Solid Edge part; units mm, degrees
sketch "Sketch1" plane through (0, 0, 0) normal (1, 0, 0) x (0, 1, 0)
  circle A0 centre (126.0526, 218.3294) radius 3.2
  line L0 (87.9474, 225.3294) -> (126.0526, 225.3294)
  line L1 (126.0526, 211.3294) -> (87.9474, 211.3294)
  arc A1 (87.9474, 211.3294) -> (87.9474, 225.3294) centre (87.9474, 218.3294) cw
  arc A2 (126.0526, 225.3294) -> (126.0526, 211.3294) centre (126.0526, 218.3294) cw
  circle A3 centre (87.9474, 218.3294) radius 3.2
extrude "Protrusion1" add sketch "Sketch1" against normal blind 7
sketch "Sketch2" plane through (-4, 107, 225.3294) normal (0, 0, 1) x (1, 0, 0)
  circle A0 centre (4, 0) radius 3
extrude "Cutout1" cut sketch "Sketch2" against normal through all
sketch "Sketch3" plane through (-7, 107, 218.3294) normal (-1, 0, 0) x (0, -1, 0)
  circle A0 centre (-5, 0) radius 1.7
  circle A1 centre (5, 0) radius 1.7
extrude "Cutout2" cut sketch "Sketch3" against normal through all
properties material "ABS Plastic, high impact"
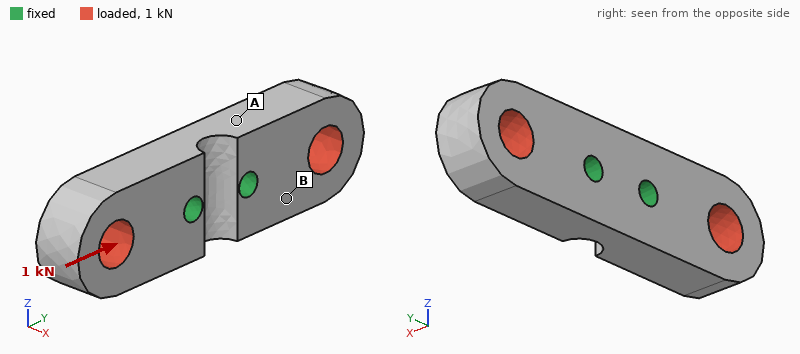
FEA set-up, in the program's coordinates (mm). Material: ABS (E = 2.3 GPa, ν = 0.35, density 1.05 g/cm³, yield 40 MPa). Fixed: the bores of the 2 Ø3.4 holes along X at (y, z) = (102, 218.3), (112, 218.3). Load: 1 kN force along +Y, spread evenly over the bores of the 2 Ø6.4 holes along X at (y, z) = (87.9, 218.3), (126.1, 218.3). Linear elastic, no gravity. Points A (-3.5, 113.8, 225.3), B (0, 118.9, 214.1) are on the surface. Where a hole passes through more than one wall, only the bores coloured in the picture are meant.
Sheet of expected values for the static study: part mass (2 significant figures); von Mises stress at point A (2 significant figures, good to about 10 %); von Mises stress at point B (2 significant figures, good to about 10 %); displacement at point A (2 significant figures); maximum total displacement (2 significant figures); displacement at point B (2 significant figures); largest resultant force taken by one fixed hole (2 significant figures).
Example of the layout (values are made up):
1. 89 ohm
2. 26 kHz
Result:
1. 4.2 g
2. 2.5 MPa
3. 5.5 MPa
4. 18 µm
5. 69 µm
6. 23 µm
7. 500 N
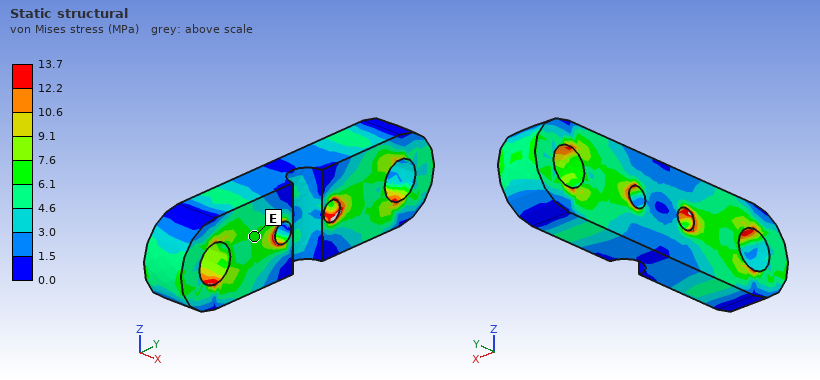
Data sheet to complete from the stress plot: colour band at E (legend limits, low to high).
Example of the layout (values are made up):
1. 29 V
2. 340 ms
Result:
1. 6.1 to 7.6 MPa
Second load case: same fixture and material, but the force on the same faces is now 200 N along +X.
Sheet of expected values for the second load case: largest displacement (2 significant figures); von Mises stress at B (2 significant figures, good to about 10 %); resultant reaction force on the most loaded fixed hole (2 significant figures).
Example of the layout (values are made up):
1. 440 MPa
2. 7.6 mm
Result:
1. 0.23 mm
2. 6.2 MPa
3. 110 N
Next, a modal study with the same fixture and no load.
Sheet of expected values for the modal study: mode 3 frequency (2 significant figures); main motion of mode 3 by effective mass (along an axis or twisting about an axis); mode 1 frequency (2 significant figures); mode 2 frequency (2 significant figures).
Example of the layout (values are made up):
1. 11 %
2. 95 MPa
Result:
1. 4800 Hz
2. twisting about X
3. 4100 Hz
4. 4100 Hz
